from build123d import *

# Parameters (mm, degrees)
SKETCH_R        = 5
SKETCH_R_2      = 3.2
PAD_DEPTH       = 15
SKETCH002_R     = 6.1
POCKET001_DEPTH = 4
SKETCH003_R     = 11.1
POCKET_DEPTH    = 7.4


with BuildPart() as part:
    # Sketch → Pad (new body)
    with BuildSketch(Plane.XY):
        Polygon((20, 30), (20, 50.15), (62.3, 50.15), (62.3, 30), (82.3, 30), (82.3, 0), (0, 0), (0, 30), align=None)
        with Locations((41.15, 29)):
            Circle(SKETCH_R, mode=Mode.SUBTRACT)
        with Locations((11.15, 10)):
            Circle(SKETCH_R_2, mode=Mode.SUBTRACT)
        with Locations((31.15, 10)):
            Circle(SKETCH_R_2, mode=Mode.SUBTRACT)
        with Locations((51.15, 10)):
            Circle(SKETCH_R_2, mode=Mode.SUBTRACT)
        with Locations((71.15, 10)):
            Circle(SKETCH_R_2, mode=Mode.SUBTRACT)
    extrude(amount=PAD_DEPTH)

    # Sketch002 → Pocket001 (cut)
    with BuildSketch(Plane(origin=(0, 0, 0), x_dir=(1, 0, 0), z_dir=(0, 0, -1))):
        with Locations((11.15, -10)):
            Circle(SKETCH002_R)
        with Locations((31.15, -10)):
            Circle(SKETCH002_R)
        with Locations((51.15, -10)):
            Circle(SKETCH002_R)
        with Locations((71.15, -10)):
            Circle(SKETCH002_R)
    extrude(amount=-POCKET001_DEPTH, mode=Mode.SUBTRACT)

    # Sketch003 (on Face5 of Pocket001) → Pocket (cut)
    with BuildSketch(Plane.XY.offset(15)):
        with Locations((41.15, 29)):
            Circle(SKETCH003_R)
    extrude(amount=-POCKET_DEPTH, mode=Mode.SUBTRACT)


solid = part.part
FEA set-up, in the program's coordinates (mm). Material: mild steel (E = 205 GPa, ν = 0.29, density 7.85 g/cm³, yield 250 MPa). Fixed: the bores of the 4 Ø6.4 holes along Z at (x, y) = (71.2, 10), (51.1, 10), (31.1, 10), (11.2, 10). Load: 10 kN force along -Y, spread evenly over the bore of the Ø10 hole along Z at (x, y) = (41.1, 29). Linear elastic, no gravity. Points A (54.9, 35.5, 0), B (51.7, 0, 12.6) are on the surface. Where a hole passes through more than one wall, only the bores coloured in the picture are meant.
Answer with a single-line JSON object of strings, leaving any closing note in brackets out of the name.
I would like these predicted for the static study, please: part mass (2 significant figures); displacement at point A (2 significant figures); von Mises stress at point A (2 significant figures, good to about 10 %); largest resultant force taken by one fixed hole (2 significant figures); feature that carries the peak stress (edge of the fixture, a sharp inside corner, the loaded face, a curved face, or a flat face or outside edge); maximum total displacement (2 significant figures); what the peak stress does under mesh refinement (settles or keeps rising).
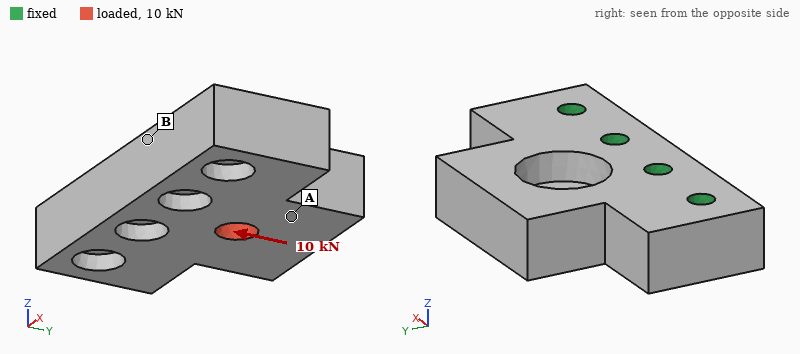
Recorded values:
{"part mass": "340 g", "displacement at point A": "6.8 µm", "von Mises stress at point A": "18 MPa", "largest resultant force taken by one fixed hole": "3.9 kN", "feature that carries the peak stress": "edge of the fixture", "maximum total displacement": "12 µm", "what the peak stress does under mesh refinement": "keeps rising"}
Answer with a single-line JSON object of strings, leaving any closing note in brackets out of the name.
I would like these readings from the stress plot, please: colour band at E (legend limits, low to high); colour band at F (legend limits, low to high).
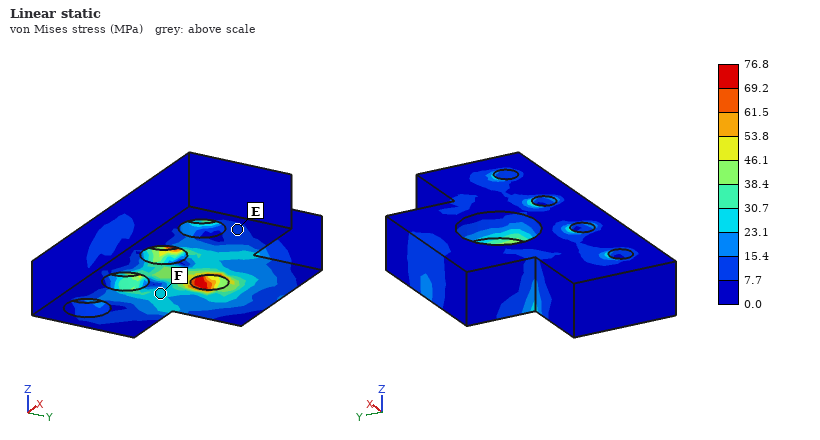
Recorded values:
{"colour band at E": "7.7 to 15.4 MPa", "colour band at F": "23.1 to 30.7 MPa"}
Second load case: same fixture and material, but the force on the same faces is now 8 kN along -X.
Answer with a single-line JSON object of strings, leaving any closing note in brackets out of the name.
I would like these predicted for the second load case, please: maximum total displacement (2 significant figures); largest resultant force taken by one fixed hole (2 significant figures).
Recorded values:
{"maximum total displacement": "5.1 µm", "largest resultant force taken by one fixed hole": "2.9 kN"}
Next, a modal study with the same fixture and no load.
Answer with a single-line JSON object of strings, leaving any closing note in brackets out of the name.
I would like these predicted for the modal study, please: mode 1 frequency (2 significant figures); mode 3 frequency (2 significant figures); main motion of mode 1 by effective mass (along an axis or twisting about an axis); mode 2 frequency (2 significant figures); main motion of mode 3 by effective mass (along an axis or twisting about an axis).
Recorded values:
{"mode 1 frequency": "6600 Hz", "mode 3 frequency": "17 kHz", "main motion of mode 1 by effective mass": "along Z", "mode 2 frequency": "13 kHz", "main motion of mode 3 by effective mass": "along X"}
